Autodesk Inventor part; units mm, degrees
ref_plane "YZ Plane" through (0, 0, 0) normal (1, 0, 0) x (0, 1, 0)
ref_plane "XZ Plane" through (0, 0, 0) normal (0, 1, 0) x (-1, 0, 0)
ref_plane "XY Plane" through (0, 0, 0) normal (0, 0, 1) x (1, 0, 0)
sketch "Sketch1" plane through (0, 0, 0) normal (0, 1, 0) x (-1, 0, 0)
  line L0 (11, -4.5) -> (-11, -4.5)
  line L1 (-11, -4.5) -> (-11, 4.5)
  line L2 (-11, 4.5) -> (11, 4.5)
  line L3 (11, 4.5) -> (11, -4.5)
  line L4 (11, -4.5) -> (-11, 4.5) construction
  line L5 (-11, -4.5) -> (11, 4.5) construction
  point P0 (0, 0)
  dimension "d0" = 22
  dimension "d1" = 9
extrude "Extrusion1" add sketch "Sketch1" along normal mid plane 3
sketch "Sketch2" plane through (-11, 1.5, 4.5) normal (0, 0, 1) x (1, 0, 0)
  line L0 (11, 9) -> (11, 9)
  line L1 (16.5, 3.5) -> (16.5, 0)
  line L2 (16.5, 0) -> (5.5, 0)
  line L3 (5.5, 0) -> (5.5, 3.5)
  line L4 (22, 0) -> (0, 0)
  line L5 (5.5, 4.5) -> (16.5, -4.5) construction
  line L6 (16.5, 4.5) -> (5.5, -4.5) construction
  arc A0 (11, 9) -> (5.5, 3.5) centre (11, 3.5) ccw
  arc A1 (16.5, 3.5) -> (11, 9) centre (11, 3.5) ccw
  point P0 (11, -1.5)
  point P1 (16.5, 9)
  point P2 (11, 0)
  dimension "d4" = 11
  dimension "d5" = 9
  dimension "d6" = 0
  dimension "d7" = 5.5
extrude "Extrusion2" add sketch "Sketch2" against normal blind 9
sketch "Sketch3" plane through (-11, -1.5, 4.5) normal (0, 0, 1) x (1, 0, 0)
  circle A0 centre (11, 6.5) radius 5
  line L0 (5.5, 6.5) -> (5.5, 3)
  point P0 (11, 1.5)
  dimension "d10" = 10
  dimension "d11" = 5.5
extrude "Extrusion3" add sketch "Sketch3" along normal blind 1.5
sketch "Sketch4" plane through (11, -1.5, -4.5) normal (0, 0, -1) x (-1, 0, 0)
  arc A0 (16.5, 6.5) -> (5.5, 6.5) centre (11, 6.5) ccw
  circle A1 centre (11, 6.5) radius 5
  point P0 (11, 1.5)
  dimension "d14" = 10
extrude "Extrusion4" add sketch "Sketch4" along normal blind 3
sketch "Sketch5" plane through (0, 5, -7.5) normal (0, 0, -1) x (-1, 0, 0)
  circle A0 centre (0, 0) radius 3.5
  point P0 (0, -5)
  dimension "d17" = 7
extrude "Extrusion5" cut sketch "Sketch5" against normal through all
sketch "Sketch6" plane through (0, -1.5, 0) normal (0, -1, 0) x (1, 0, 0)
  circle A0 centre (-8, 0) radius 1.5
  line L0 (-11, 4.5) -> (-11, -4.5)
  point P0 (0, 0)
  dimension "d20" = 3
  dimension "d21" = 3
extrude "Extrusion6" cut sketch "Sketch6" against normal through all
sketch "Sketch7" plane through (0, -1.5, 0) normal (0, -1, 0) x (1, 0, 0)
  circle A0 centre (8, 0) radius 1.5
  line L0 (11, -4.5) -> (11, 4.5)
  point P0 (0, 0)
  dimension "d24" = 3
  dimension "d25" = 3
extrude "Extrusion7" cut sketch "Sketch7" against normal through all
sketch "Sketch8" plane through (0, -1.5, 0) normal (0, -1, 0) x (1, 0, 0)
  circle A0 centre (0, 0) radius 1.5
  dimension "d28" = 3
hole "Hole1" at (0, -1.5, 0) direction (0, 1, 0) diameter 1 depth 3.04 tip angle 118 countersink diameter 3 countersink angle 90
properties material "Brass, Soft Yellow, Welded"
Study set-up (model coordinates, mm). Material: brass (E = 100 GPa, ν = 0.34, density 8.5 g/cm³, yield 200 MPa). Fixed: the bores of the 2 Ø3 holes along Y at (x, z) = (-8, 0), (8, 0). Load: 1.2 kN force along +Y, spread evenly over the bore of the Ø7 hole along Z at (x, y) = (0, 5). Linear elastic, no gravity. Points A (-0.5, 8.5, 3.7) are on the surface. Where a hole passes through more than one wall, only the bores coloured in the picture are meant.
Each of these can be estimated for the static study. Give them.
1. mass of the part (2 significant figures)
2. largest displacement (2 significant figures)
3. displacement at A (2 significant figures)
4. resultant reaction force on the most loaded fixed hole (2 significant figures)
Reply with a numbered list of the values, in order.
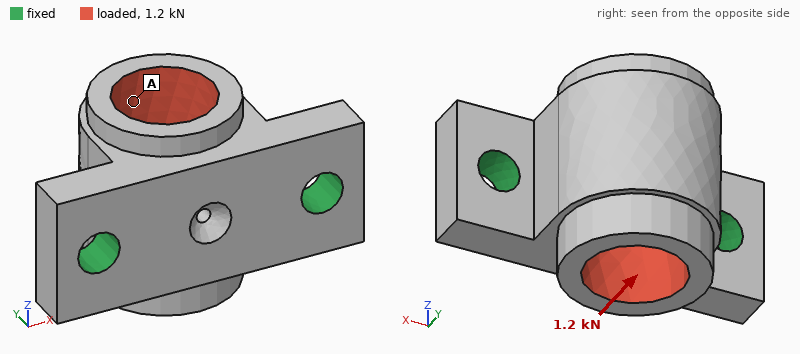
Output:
1. 9.8 g
2. 10 µm
3. 4.8 µm
4. 620 N
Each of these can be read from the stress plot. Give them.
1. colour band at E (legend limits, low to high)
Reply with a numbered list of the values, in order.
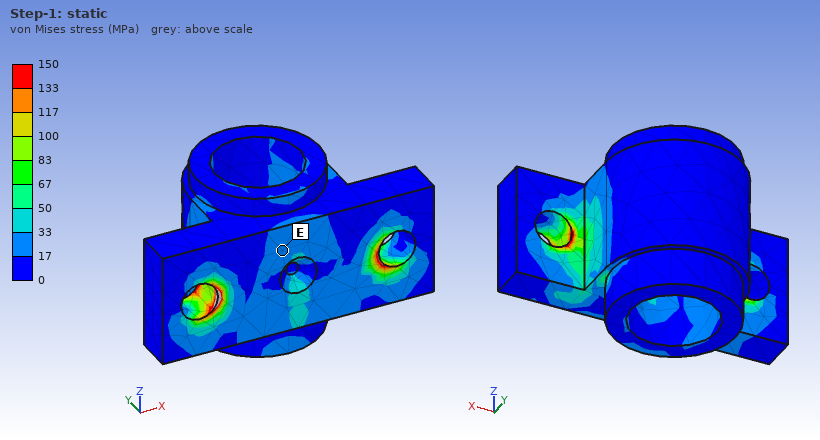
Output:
1. 17 to 33 MPa
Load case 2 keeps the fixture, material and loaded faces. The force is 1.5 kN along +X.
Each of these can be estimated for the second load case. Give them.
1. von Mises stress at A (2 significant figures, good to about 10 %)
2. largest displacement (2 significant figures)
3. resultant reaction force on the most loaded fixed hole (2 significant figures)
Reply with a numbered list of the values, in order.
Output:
1. 25 MPa
2. 18 µm
3. 940 N
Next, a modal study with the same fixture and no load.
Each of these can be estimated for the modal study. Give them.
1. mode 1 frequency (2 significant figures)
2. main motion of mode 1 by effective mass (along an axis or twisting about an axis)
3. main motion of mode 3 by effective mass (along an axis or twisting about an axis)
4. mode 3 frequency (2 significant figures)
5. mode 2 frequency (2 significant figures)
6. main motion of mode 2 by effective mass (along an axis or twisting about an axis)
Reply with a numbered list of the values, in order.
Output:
1. 13 kHz
2. along Z
3. along Y
4. 30 kHz
5. 21 kHz
6. along X
